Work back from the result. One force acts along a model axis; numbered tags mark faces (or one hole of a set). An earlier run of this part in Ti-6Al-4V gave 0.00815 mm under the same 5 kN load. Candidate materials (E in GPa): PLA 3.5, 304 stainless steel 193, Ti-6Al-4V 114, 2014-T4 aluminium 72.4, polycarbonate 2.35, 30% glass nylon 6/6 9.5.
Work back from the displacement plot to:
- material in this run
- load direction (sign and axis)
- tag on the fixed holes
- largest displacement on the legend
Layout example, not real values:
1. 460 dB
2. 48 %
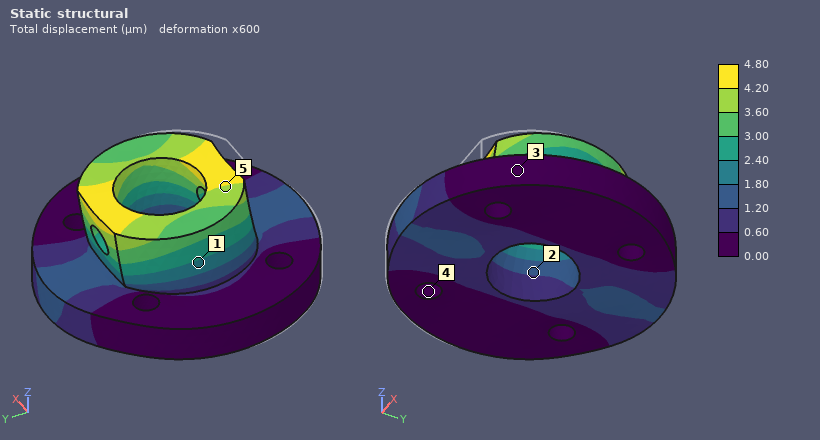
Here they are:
1. 304 stainless steel
2. +Y
3. 4
4. 4.80 µm
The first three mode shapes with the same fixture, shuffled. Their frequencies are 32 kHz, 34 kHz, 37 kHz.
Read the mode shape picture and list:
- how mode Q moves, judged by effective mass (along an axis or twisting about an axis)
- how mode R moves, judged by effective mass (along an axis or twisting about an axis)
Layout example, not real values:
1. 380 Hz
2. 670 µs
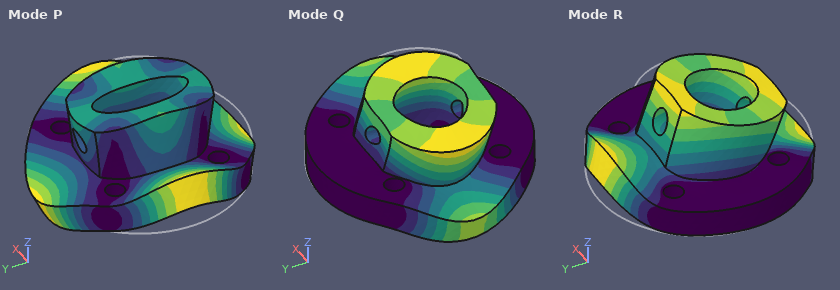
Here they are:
1. along X
2. along Y
